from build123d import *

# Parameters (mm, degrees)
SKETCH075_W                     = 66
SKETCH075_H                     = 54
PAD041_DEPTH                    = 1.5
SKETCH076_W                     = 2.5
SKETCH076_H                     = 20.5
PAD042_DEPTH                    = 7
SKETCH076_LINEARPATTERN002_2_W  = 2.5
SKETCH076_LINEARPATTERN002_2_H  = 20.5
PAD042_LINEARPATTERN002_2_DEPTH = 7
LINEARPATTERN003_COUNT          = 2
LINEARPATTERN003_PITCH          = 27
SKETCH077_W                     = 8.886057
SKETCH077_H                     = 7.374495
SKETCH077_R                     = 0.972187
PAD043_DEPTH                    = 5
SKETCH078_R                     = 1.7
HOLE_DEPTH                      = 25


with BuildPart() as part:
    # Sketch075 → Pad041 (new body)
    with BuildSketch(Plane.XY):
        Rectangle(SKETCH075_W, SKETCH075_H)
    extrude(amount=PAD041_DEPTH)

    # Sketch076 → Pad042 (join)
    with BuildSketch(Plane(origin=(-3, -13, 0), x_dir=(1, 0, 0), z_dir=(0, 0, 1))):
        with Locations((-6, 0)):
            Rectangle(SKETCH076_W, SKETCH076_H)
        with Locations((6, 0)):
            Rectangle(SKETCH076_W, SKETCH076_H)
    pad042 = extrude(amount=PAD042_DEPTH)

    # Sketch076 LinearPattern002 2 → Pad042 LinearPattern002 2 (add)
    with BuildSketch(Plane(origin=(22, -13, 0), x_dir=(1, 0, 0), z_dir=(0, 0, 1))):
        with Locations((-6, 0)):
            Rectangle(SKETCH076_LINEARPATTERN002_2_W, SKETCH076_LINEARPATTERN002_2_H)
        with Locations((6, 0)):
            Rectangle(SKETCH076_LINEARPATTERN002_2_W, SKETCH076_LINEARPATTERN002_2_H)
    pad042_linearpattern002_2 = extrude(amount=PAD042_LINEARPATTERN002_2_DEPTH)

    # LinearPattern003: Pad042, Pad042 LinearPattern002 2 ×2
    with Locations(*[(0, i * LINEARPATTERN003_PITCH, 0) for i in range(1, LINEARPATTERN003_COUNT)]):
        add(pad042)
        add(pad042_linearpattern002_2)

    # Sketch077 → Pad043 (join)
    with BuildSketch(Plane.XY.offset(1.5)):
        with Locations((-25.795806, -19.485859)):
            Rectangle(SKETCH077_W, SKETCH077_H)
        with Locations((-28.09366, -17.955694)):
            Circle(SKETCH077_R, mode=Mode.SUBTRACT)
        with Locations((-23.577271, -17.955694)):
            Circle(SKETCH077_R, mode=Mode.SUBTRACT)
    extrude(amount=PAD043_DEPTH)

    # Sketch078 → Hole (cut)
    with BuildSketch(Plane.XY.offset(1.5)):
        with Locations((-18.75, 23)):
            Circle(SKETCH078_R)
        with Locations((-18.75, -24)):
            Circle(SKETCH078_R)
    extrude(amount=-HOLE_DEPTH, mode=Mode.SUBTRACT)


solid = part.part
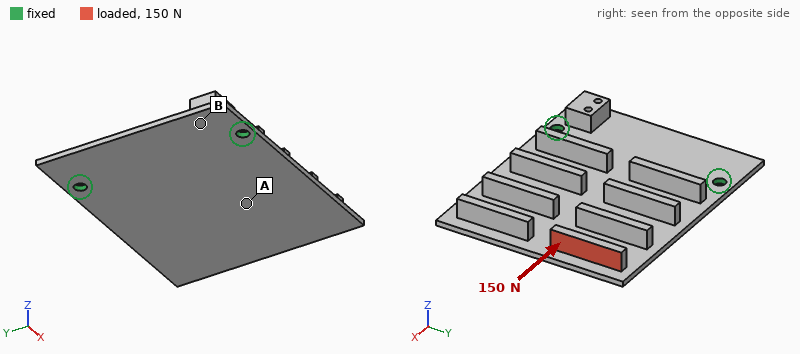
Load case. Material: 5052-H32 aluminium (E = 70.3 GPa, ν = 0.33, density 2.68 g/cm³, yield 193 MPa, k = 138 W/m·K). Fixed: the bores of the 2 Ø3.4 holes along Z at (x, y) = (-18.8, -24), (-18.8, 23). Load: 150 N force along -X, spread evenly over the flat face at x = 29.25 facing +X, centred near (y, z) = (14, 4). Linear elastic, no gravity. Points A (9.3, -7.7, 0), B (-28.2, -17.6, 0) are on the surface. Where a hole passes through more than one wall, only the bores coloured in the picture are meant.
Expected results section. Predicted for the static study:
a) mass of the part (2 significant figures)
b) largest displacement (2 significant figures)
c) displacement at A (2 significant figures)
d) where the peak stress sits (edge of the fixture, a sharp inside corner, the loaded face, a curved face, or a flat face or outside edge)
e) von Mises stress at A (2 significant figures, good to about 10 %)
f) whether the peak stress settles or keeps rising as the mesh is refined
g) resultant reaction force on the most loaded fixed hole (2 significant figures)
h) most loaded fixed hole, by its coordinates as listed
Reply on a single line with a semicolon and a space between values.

21 g; 0.68 mm; 0.21 mm; edge of the fixture; 20 MPa; keeps rising; 120 N; (-18.8, 23)
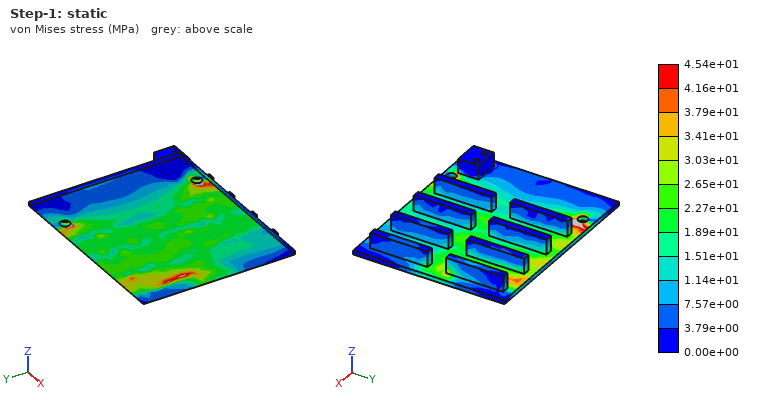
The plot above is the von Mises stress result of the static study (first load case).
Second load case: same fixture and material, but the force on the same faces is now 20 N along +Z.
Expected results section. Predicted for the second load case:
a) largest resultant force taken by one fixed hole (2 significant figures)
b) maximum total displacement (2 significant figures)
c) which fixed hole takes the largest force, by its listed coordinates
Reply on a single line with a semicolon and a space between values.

18 N; 0.88 mm; (-18.8, 23)
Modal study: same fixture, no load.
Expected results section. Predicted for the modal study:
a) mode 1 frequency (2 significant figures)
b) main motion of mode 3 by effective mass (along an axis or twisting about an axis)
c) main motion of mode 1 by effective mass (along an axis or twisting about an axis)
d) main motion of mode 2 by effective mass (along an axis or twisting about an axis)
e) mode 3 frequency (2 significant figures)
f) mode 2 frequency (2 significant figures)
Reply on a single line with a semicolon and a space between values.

350 Hz; along Z; along Z; twisting about X; 2200 Hz; 1200 Hz
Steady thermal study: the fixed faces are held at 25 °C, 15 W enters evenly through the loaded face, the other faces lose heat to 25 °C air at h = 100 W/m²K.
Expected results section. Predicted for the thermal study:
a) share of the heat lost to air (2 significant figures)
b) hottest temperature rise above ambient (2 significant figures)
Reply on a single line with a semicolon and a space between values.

77 %; 50 K
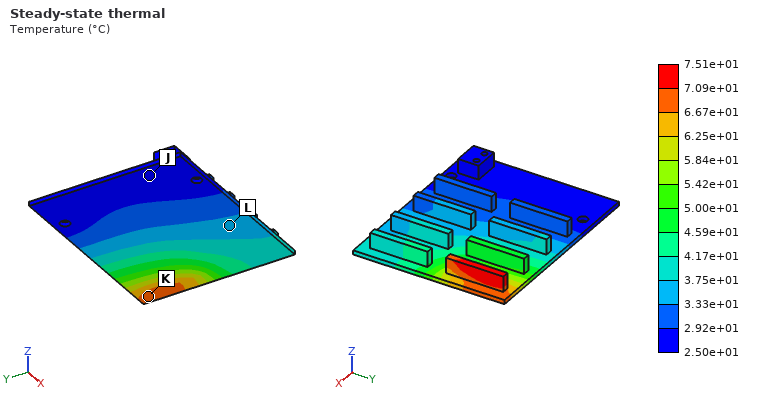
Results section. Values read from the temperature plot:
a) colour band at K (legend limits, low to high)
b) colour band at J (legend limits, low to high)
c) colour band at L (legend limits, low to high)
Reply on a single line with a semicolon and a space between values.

6.67e+01 to 7.09e+01 °C; 2.50e+01 to 2.92e+01 °C; 3.33e+01 to 3.75e+01 °C
